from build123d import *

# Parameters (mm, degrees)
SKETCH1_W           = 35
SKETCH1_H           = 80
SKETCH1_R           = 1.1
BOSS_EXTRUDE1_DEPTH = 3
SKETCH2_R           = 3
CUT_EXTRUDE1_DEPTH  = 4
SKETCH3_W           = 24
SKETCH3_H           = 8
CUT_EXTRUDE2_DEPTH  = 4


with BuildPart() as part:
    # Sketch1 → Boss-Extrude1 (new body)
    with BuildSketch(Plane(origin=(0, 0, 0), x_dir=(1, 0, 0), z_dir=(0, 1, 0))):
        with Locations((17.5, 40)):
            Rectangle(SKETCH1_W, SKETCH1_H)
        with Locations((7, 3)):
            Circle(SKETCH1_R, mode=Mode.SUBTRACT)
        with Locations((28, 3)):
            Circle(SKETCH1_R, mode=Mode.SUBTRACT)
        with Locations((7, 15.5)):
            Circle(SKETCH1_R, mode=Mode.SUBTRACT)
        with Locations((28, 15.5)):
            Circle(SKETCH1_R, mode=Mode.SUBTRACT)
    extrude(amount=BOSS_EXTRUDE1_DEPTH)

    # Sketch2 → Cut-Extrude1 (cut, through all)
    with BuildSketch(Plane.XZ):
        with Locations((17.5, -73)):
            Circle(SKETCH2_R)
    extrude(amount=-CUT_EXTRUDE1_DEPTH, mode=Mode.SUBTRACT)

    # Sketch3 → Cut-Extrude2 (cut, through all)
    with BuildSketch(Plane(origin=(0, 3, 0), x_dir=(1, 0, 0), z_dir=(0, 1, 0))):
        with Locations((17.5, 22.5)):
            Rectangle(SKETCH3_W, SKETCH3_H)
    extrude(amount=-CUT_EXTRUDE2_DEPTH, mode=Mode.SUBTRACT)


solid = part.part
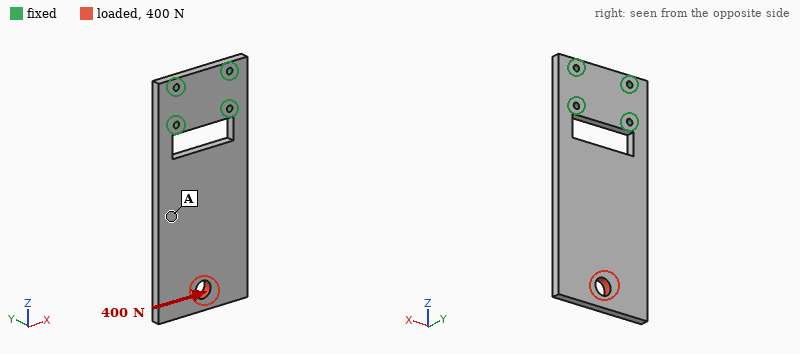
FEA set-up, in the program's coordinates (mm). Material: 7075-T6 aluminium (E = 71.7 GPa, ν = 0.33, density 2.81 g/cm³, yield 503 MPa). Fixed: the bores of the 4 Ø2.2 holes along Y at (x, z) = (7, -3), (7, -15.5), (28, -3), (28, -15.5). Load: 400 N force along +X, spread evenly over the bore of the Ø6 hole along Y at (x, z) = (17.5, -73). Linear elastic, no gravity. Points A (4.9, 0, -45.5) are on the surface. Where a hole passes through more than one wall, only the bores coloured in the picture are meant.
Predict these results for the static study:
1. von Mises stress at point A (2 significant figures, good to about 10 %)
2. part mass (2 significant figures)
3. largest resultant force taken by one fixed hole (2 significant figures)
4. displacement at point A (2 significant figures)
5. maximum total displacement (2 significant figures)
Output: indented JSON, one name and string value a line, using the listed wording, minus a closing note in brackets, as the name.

{
  "von Mises stress at point A": "14 MPa",
  "part mass": "22 g",
  "largest resultant force taken by one fixed hole": "610 N",
  "displacement at point A": "0.052 mm",
  "maximum total displacement": "0.10 mm"
}
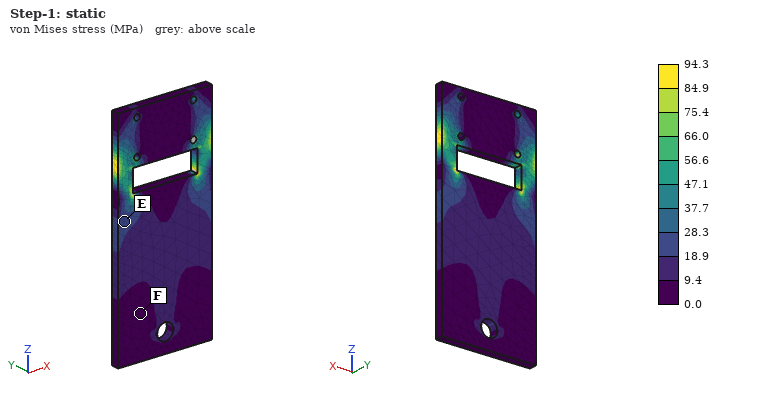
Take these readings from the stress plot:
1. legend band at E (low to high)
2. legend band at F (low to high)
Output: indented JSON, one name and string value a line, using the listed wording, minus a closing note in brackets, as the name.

{
  "legend band at E": "18.9 to 28.3 MPa",
  "legend band at F": "0.0 to 9.4 MPa"
}
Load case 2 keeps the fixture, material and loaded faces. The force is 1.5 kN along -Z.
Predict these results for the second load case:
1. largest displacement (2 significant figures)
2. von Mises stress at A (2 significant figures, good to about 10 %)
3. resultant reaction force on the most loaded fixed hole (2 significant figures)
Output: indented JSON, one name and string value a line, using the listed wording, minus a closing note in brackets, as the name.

{
  "largest displacement": "30 µm",
  "von Mises stress at A": "18 MPa",
  "resultant reaction force on the most loaded fixed hole": "560 N"
}
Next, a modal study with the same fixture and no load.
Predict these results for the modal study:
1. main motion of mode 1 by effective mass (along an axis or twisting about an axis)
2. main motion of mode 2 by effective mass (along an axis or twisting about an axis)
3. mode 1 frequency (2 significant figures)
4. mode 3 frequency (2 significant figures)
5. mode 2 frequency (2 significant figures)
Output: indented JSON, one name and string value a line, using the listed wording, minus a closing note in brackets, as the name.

{
  "main motion of mode 1 by effective mass": "along Y",
  "main motion of mode 2 by effective mass": "twisting about Z",
  "mode 1 frequency": "380 Hz",
  "mode 3 frequency": "3100 Hz",
  "mode 2 frequency": "2000 Hz"
}
